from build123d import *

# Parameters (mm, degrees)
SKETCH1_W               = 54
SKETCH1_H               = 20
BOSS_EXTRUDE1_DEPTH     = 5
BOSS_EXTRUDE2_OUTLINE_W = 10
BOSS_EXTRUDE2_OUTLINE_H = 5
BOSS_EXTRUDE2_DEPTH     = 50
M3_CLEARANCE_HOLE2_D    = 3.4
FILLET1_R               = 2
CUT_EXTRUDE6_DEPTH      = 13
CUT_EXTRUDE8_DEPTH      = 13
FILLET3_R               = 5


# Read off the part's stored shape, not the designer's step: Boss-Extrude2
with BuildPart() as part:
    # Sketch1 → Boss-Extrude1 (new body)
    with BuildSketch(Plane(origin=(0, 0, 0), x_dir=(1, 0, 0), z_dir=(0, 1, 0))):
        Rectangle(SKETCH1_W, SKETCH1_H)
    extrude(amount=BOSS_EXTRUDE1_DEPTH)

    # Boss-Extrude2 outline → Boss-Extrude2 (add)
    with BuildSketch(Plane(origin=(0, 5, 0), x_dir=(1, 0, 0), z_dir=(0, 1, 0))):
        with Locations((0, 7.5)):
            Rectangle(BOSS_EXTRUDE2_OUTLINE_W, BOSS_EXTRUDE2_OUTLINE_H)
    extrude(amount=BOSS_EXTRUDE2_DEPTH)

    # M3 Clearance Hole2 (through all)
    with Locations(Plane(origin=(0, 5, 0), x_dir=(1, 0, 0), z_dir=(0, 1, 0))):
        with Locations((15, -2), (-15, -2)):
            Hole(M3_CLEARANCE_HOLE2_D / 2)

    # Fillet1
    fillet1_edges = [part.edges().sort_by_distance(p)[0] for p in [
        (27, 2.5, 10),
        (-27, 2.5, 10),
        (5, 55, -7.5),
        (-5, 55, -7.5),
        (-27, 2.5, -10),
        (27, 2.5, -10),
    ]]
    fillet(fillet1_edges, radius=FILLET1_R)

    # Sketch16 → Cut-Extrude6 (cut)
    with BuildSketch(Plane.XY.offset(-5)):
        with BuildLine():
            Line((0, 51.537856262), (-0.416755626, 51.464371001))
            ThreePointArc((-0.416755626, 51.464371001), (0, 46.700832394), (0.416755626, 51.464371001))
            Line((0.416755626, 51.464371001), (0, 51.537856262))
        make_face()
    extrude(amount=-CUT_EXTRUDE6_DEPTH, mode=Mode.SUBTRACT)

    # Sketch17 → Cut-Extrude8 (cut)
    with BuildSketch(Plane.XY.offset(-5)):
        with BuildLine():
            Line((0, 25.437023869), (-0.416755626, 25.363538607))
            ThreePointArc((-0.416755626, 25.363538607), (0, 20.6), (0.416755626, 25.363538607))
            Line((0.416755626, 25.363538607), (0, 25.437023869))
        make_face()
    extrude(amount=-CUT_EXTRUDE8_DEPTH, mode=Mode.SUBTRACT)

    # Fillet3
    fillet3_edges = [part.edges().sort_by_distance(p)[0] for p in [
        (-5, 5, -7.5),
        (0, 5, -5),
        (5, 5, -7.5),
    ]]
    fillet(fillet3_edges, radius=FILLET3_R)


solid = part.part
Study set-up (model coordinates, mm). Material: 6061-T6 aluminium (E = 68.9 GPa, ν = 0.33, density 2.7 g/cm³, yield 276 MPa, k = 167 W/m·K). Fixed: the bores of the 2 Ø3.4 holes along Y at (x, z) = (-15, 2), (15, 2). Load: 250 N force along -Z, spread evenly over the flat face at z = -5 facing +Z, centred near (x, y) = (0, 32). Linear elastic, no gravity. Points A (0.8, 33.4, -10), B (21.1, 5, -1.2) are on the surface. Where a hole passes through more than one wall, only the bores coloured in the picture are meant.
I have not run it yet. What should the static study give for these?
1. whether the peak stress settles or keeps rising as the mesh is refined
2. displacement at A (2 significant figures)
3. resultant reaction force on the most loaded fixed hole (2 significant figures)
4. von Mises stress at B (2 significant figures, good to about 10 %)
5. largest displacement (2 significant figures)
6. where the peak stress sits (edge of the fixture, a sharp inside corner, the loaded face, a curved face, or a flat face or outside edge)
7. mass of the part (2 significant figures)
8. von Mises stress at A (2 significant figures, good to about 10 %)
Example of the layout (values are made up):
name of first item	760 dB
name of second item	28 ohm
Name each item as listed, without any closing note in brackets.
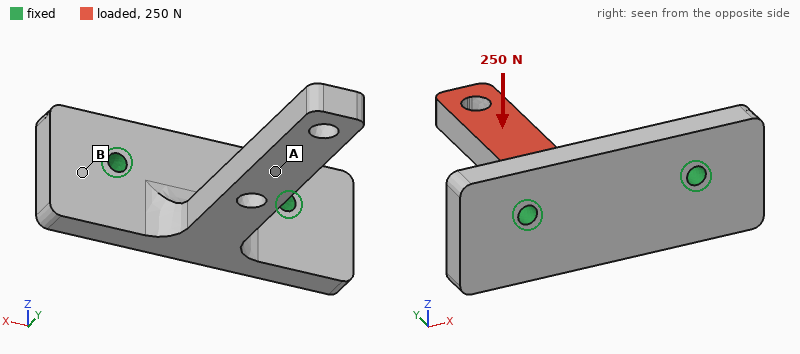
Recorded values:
whether the peak stress settles or keeps rising as the mesh is refined	keeps rising
displacement at A	0.35 mm
resultant reaction force on the most loaded fixed hole	130 N
von Mises stress at B	14 MPa
largest displacement	0.77 mm
where the peak stress sits	a sharp inside corner
mass of the part	21 g
von Mises stress at A	29 MPa
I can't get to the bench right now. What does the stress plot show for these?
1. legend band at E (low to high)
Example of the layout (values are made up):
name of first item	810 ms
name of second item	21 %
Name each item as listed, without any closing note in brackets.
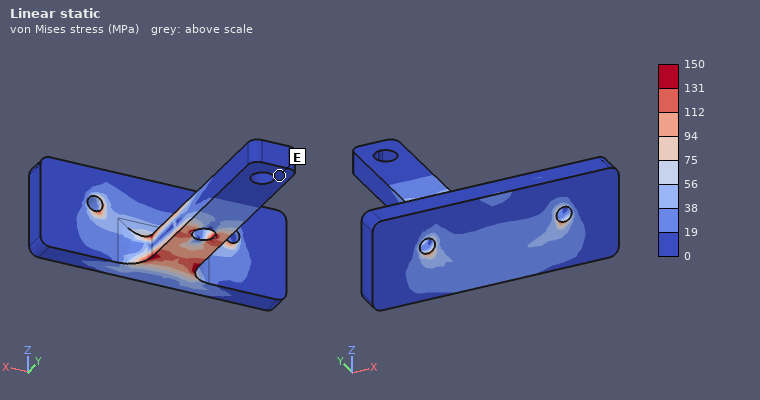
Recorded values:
legend band at E	0 to 19 MPa
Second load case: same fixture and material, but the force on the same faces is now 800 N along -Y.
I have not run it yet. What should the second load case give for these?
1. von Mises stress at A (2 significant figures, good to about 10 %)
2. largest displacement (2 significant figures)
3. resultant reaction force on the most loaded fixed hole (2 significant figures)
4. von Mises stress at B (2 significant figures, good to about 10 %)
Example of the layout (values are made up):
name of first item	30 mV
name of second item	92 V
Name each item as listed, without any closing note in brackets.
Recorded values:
von Mises stress at A	16 MPa
largest displacement	0.20 mm
resultant reaction force on the most loaded fixed hole	410 N
von Mises stress at B	10 MPa
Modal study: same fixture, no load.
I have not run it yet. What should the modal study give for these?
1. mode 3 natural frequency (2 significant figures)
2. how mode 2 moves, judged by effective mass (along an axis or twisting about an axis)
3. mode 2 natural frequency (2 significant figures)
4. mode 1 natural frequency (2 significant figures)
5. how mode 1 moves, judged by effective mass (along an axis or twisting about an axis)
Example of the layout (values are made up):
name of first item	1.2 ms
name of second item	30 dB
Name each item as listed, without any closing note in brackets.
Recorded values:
mode 3 natural frequency	7900 Hz
how mode 2 moves, judged by effective mass	along X
mode 2 natural frequency	3000 Hz
mode 1 natural frequency	1500 Hz
how mode 1 moves, judged by effective mass	along Z
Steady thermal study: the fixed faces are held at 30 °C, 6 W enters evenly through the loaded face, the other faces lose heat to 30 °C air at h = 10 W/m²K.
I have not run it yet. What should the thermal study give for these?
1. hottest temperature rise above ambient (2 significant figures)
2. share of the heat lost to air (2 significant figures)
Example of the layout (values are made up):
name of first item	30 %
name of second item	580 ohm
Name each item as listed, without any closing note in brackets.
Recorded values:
hottest temperature rise above ambient	24 K
share of the heat lost to air	3.8 %
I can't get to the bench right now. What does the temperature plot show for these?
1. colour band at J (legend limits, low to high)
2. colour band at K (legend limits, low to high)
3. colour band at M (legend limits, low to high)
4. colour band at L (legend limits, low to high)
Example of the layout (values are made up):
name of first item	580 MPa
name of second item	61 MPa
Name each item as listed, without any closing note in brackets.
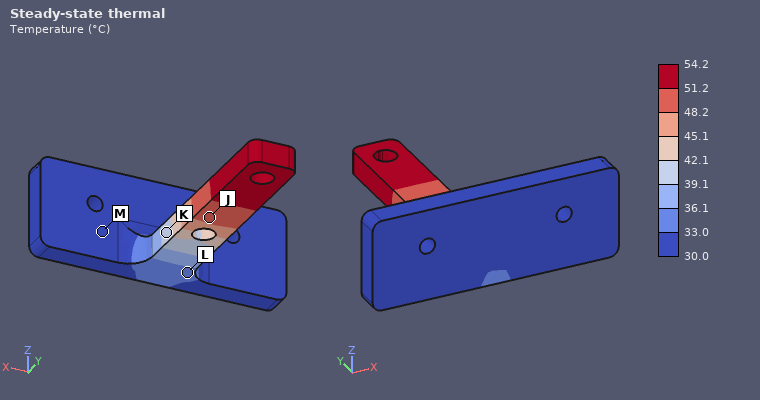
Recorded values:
colour band at J	48.2 to 51.2 °C
colour band at K	39.1 to 42.1 °C
colour band at M	30.0 to 33.0 °C
colour band at L	33.0 to 36.1 °C
